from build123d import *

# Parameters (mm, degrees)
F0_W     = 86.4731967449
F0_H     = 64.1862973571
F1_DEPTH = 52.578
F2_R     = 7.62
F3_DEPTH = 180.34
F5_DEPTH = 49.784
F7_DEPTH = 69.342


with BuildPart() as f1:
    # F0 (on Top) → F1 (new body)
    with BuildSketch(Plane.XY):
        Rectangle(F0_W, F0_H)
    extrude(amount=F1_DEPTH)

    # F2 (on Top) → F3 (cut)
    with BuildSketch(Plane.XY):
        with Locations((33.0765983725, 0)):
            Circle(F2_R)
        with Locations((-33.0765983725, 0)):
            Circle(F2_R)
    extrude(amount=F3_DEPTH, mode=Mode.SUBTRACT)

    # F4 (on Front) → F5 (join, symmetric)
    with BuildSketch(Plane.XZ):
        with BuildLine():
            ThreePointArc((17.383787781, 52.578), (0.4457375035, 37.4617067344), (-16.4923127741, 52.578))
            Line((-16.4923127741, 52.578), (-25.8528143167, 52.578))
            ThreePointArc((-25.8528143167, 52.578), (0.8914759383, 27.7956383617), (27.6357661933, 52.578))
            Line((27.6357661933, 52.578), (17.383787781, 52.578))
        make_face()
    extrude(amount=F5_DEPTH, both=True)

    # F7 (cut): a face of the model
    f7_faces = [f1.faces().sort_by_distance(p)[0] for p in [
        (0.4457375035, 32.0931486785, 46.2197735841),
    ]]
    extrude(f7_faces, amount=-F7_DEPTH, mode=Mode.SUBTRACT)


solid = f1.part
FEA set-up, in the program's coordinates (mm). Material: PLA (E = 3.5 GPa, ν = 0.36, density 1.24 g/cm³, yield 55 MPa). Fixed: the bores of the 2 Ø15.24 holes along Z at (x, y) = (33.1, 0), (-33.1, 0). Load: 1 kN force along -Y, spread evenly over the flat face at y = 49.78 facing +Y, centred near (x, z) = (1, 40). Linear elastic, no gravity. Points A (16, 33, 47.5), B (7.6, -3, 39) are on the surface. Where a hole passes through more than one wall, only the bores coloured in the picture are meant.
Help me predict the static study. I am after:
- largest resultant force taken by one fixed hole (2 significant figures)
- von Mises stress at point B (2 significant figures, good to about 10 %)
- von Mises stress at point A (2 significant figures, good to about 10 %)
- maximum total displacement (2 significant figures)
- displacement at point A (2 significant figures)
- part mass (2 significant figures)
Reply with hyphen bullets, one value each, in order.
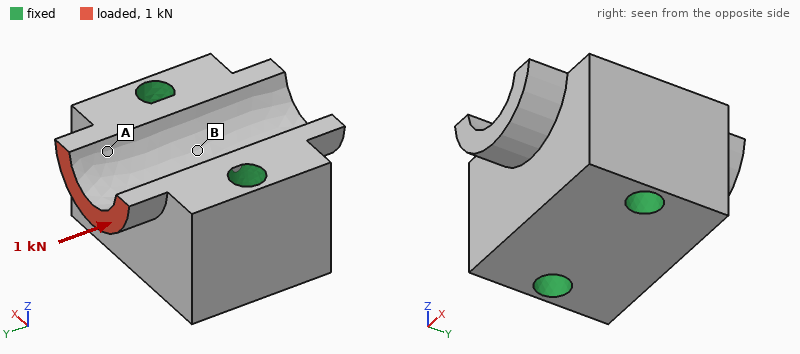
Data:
- 540 N
- 0.29 MPa
- 1.2 MPa
- 24 µm
- 13 µm
- 330 g
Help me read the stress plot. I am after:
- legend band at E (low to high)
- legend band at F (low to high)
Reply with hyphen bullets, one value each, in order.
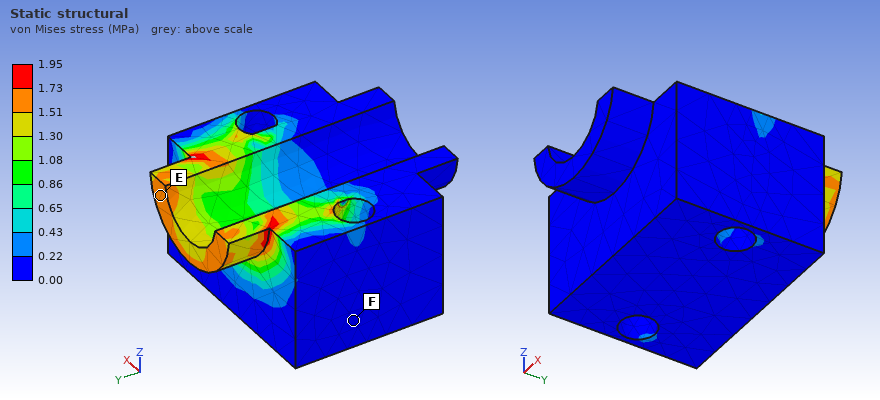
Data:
- 1.51 to 1.73 MPa
- 0.00 to 0.22 MPa
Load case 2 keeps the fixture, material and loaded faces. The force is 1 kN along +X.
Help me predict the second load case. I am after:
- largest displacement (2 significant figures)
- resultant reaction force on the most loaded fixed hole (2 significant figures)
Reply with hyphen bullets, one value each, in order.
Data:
- 0.15 mm
- 840 N
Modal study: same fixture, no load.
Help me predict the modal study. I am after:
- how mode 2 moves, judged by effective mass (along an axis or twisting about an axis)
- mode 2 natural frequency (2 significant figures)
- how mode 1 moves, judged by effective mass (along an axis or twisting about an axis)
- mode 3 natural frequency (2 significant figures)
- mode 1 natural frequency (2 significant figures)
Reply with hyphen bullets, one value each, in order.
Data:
- along Z
- 4900 Hz
- twisting about X
- 5100 Hz
- 4700 Hz
